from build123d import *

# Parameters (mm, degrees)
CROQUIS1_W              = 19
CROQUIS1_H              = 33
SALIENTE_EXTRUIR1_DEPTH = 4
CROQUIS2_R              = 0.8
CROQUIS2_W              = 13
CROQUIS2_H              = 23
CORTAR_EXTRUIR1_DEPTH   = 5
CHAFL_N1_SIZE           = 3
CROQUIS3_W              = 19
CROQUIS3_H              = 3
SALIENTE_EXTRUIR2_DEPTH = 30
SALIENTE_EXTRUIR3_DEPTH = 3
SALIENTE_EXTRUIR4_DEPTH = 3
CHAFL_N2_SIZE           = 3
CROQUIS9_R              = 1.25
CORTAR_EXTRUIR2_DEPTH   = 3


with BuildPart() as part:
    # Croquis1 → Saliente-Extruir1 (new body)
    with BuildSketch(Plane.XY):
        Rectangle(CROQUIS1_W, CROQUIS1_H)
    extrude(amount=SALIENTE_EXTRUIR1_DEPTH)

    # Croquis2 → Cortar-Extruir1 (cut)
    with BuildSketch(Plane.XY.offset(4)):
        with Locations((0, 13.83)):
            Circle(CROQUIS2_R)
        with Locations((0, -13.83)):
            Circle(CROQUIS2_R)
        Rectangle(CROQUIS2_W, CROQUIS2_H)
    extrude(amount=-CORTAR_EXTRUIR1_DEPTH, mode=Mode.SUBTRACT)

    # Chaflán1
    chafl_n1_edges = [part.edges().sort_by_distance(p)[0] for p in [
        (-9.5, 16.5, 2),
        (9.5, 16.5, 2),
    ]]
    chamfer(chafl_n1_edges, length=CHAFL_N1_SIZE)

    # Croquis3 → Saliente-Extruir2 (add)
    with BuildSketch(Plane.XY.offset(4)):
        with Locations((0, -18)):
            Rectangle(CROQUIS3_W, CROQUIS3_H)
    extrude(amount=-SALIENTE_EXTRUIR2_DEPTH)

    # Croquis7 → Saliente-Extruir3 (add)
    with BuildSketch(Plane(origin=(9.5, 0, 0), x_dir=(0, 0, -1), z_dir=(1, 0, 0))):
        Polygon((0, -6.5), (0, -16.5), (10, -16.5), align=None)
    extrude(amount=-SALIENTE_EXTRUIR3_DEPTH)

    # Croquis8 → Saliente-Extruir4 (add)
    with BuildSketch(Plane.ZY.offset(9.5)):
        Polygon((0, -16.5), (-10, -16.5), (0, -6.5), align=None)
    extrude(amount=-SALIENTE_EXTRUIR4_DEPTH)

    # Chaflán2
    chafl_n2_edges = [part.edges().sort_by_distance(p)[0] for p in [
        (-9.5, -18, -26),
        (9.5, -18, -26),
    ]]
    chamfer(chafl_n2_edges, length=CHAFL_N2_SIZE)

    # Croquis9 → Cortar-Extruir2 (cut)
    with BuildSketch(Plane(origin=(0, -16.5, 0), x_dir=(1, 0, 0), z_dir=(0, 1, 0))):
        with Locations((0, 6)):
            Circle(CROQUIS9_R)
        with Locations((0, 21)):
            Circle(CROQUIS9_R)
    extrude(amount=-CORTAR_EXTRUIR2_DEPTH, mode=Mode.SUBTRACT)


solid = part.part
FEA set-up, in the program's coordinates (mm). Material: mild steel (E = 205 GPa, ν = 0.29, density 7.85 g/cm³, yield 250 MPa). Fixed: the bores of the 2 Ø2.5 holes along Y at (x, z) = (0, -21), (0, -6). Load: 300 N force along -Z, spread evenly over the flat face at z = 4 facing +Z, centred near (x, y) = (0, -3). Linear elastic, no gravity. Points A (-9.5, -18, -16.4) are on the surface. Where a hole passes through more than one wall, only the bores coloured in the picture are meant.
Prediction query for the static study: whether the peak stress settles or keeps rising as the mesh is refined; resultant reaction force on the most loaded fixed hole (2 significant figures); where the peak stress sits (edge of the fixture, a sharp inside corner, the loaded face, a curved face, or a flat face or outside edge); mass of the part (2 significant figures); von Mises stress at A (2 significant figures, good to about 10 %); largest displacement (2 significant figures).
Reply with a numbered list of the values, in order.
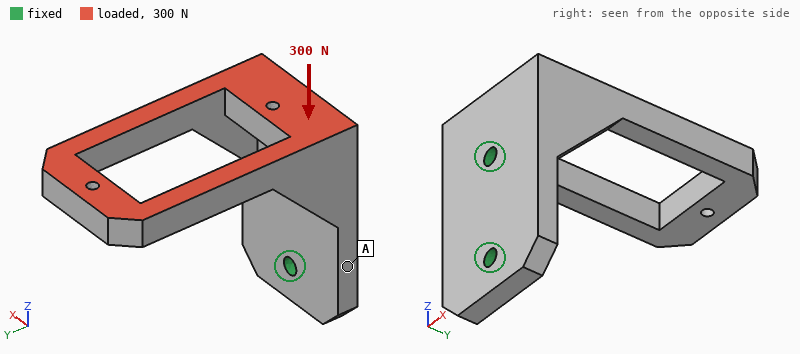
1. keeps rising
2. 230 N
3. edge of the fixture
4. 25 g
5. 17 MPa
6. 0.12 mm
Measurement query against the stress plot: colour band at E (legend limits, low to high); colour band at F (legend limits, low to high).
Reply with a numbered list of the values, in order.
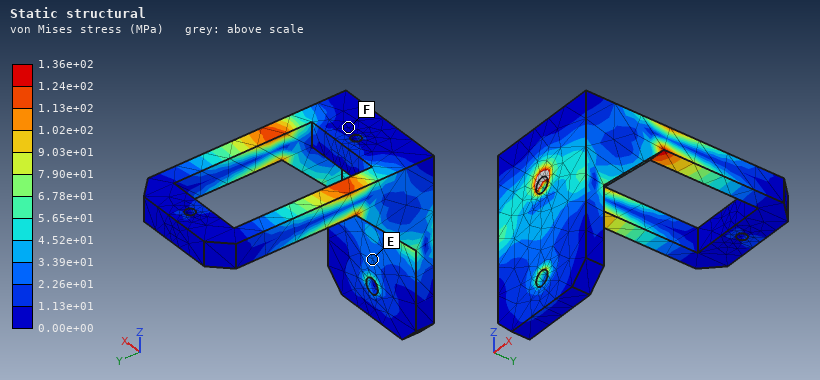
1. 2.26e+01 to 3.39e+01 MPa
2. 0.00e+00 to 1.13e+01 MPa
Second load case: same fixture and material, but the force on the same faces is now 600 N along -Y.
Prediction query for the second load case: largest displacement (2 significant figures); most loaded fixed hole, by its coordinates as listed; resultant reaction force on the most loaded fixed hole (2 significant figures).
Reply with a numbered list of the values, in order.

1. 89 µm
2. (0, -6)
3. 800 N
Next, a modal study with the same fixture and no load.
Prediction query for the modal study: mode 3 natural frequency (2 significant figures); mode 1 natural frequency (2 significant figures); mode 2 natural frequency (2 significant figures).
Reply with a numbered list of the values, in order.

1. 7600 Hz
2. 2600 Hz
3. 2700 Hz
